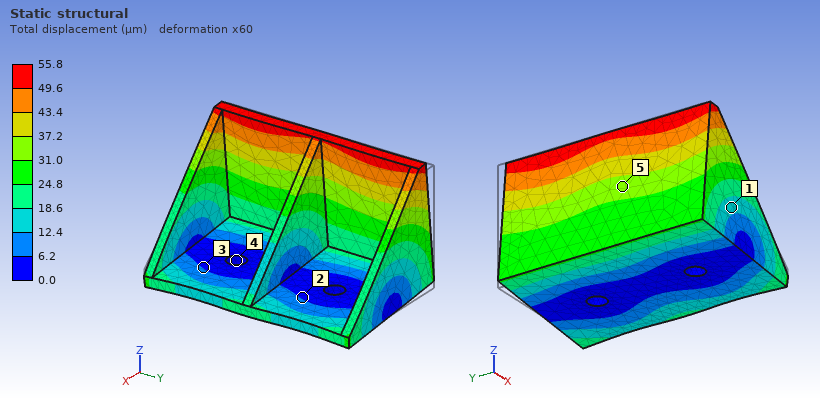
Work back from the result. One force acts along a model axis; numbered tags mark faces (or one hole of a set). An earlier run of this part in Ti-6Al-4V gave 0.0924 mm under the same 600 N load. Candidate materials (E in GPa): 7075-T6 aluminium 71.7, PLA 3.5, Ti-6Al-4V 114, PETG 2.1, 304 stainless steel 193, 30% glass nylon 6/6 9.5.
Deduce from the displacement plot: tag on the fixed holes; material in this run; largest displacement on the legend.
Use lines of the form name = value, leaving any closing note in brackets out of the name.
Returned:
tag on the fixed holes = 4
material in this run = 304 stainless steel
largest displacement on the legend = 55.8 µm
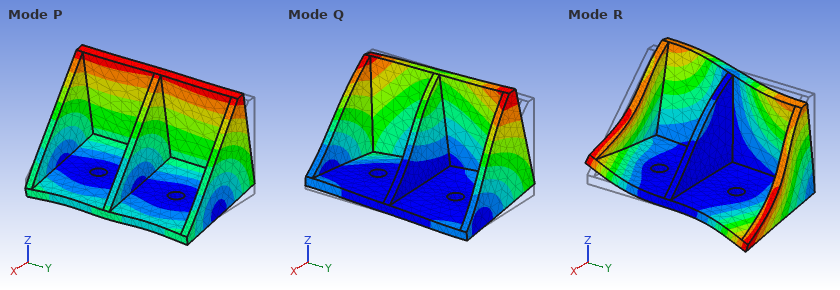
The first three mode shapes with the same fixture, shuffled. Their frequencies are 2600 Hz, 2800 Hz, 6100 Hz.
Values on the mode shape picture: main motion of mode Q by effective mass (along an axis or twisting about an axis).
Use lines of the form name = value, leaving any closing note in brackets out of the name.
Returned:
main motion of mode Q by effective mass = along Y
